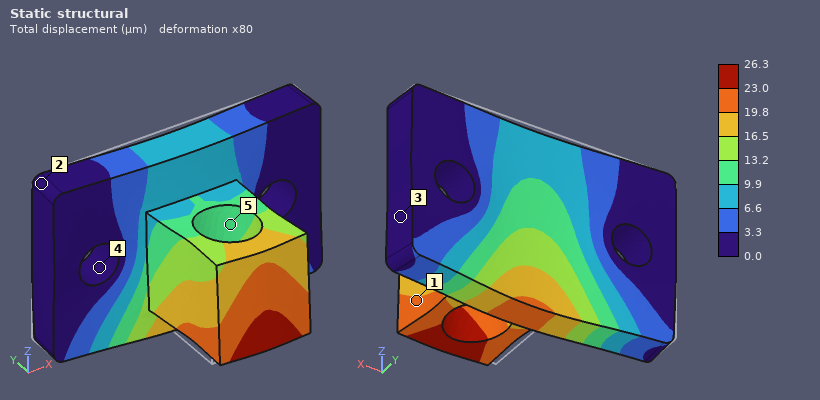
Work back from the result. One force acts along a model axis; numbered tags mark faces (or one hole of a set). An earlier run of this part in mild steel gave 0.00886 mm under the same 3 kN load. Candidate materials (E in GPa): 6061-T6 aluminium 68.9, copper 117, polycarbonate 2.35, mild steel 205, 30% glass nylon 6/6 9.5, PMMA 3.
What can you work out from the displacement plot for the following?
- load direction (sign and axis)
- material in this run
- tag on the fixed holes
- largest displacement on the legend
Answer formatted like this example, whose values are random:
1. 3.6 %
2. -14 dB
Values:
1. -Y
2. 6061-T6 aluminium
3. 4
4. 26.3 µm
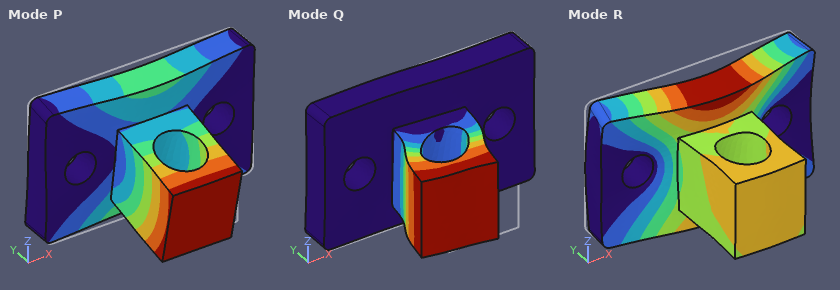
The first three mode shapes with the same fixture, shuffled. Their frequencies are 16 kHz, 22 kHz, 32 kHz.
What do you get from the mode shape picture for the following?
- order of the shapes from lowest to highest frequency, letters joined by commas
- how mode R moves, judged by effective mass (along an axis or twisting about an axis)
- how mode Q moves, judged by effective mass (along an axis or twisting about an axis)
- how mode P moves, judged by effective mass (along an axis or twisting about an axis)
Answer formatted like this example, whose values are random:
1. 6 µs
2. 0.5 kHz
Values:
1. P, Q, R
2. along Y
3. along X
4. along Z
